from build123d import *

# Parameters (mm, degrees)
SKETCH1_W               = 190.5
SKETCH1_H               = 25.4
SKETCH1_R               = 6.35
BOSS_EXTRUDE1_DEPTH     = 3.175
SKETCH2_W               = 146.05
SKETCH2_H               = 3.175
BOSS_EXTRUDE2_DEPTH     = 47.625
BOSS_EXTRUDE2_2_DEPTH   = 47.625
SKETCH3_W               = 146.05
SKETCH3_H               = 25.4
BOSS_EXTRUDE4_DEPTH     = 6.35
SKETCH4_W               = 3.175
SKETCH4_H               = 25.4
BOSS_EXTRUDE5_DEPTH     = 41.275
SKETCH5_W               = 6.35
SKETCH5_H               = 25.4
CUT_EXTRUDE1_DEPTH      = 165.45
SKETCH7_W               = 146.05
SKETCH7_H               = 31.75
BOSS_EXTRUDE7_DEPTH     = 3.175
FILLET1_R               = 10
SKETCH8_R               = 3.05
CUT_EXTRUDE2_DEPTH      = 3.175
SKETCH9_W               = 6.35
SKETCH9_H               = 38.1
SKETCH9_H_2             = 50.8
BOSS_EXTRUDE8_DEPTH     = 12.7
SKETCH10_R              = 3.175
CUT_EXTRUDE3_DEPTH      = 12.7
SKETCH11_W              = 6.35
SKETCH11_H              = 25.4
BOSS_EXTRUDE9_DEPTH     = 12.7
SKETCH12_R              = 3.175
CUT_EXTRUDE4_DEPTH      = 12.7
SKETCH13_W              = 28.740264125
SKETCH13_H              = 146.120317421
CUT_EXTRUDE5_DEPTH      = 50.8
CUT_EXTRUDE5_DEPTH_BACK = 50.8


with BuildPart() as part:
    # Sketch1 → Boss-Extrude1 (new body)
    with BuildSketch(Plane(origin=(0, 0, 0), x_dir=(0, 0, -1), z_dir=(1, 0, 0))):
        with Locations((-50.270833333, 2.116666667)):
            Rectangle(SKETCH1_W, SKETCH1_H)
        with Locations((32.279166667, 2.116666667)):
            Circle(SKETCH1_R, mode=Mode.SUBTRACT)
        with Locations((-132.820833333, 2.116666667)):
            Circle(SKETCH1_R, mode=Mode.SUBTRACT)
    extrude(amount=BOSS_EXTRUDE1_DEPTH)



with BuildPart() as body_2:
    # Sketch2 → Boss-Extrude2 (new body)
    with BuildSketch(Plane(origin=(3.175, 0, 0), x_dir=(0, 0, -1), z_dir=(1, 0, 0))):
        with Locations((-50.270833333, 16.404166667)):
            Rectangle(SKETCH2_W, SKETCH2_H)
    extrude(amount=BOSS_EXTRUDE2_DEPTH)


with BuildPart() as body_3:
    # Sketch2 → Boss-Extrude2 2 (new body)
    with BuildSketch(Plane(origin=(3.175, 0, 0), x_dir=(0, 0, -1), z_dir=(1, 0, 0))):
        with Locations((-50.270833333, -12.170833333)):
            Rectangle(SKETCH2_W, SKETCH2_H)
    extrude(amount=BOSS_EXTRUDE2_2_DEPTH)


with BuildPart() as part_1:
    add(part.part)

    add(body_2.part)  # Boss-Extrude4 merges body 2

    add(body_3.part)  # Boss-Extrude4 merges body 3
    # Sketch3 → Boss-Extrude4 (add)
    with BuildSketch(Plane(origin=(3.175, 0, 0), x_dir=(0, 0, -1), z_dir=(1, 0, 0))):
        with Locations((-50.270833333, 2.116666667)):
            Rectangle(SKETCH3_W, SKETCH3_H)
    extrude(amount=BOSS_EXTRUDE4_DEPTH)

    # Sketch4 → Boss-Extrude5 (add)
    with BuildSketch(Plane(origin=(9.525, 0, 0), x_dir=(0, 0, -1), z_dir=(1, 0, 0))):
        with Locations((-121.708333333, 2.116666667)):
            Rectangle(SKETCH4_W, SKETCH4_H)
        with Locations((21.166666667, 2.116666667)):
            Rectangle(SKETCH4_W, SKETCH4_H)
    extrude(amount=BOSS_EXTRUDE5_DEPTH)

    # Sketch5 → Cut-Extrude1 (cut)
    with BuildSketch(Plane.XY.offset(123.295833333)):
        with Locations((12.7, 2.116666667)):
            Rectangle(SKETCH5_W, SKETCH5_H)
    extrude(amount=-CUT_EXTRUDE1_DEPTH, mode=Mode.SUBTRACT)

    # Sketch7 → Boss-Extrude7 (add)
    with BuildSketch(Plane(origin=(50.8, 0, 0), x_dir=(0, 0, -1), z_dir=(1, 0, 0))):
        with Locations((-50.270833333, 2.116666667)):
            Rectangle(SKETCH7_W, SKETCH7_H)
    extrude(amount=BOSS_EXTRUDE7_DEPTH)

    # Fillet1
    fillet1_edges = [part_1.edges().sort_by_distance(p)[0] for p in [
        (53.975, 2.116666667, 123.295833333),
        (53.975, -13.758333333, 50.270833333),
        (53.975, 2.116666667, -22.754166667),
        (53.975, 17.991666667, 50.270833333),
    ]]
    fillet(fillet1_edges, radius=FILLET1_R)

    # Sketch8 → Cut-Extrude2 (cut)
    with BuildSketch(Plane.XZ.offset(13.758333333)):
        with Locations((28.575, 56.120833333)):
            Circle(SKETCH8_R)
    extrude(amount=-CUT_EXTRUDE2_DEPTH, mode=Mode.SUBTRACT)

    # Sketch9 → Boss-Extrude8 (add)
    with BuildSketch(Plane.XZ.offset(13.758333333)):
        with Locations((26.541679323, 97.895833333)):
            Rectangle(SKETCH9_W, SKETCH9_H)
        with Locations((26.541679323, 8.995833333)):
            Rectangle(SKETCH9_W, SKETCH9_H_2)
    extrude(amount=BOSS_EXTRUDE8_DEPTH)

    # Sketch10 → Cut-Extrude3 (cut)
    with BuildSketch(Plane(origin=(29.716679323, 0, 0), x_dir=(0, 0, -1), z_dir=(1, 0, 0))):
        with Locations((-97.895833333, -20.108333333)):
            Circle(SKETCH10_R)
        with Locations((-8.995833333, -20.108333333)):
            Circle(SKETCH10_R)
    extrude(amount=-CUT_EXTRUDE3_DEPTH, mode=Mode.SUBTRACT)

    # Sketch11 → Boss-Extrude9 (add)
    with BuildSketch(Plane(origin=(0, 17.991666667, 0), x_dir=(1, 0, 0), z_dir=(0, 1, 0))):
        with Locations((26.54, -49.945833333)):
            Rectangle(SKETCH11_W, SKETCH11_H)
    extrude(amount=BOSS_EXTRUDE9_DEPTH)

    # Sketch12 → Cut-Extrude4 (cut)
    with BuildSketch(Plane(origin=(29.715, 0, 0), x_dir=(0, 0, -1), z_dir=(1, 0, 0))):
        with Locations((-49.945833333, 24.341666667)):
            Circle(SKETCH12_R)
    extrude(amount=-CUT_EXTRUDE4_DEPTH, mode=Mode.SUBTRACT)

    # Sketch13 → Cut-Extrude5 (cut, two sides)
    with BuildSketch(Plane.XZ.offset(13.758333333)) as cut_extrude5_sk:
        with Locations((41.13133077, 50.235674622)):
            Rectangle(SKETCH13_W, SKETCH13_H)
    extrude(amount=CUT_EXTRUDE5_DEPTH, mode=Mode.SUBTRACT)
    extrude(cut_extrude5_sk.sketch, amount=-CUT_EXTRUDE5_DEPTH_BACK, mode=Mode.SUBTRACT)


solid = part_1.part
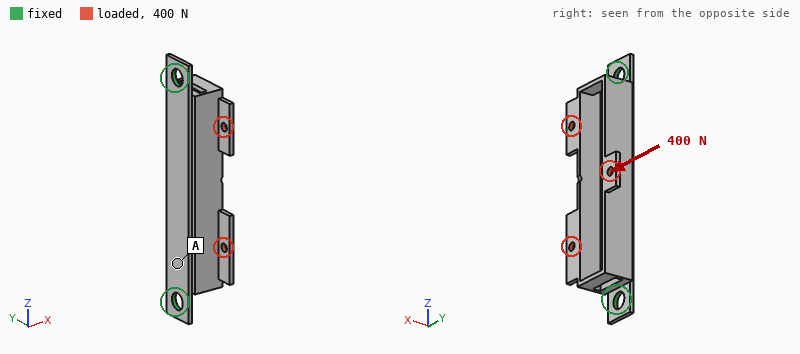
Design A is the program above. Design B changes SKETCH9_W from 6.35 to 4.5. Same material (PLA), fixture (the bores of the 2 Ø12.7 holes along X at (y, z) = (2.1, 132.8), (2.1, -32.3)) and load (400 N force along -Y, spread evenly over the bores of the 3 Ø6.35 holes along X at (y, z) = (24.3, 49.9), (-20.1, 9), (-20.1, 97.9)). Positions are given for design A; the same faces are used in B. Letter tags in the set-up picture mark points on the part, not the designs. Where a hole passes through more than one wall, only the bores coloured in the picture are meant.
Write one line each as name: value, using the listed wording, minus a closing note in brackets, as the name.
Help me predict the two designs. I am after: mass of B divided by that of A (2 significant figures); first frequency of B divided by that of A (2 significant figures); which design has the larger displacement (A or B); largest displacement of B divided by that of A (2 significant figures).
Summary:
mass of B divided by that of A: 0.99
first frequency of B divided by that of A: 1.0
which design has the larger displacement: B
largest displacement of B divided by that of A: 1.1
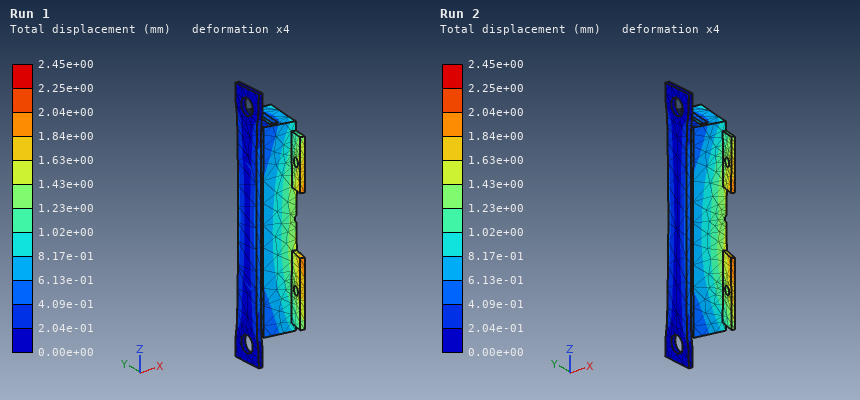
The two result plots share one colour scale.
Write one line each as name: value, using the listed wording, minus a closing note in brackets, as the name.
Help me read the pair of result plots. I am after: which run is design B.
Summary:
which run is design B: Run 2
